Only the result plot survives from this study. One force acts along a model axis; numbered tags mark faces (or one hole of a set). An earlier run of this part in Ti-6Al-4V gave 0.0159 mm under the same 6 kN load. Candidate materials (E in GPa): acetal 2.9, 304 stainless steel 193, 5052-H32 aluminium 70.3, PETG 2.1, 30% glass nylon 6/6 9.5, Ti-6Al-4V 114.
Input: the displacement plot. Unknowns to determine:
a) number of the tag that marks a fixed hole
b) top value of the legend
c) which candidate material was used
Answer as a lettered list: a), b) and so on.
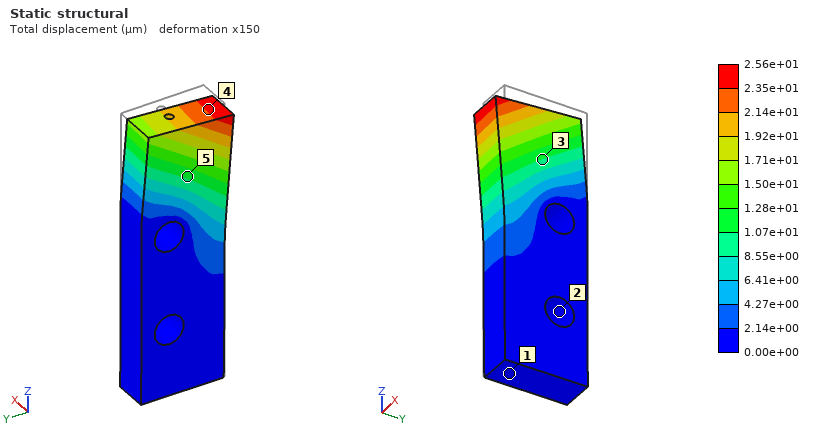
a) 2
b) 2.56e+01 µm
c) 5052-H32 aluminium
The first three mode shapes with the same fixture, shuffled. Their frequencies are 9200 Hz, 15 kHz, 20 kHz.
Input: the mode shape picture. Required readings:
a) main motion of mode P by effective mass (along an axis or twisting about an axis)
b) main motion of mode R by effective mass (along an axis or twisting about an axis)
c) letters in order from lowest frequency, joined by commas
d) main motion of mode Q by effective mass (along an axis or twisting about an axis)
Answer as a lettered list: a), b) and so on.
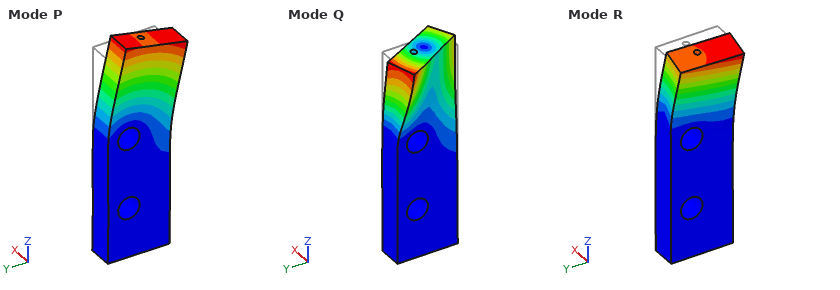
a) along Y
b) along X
c) R, P, Q
d) twisting about Z
